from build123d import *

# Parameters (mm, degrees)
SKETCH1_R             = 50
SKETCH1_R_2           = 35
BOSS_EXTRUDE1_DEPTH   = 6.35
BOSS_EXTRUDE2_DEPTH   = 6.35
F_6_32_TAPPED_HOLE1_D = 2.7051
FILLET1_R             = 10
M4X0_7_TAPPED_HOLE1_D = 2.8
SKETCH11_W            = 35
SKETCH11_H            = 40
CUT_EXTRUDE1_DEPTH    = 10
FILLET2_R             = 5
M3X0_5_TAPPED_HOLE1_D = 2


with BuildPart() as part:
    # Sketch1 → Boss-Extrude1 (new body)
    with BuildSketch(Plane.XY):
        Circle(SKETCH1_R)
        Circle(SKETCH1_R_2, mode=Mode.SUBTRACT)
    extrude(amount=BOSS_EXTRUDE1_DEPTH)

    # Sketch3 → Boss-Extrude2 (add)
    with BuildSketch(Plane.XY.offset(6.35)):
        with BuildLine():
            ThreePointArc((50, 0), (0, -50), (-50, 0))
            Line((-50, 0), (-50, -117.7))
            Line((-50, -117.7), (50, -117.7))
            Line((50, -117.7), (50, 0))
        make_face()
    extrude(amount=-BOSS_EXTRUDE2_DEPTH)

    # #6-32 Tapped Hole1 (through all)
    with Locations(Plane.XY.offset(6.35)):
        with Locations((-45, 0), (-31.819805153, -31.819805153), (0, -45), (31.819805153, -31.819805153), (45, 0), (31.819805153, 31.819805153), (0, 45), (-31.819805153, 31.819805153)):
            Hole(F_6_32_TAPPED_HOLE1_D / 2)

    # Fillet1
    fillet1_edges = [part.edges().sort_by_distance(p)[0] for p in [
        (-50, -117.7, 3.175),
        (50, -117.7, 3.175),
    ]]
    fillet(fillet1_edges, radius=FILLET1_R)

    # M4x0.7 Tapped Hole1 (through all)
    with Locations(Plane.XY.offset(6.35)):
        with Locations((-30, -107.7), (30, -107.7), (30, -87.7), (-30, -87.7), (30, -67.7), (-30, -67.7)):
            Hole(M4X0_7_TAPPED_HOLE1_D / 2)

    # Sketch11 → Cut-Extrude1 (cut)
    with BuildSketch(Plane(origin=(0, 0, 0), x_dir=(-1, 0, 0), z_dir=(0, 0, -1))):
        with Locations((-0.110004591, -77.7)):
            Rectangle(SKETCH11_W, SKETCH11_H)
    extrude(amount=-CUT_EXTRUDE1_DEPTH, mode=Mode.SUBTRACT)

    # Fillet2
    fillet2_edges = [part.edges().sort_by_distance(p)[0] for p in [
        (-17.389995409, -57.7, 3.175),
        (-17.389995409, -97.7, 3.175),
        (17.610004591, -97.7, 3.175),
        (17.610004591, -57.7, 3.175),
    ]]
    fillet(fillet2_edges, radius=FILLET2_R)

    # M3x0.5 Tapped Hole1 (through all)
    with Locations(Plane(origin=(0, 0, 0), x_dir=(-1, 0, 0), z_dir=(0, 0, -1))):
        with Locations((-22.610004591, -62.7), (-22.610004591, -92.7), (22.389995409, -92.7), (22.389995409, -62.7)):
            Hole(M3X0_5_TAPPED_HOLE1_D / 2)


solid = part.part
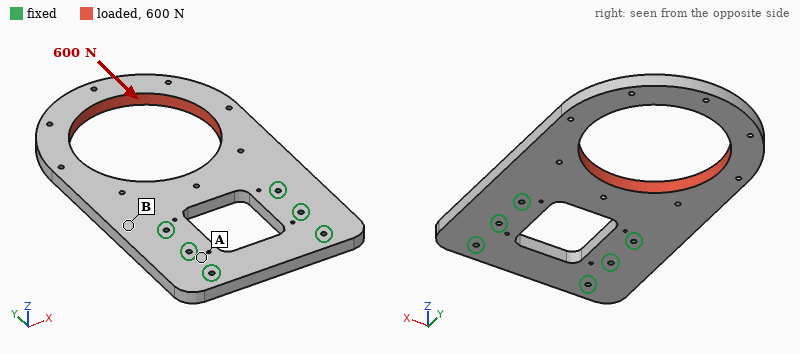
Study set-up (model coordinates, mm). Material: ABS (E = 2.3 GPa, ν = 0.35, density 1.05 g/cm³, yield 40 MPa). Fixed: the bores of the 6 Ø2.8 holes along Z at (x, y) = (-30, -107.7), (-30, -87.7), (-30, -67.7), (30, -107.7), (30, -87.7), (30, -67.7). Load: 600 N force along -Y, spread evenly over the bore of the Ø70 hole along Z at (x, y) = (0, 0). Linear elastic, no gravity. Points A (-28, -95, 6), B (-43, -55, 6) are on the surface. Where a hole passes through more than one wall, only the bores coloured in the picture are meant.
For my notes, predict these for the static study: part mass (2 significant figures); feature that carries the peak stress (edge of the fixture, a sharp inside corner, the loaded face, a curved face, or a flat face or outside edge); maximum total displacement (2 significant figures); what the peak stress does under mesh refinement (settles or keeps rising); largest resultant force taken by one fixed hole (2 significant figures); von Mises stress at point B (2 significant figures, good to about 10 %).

69 g
edge of the fixture
0.19 mm
keeps rising
200 N
1.7 MPa
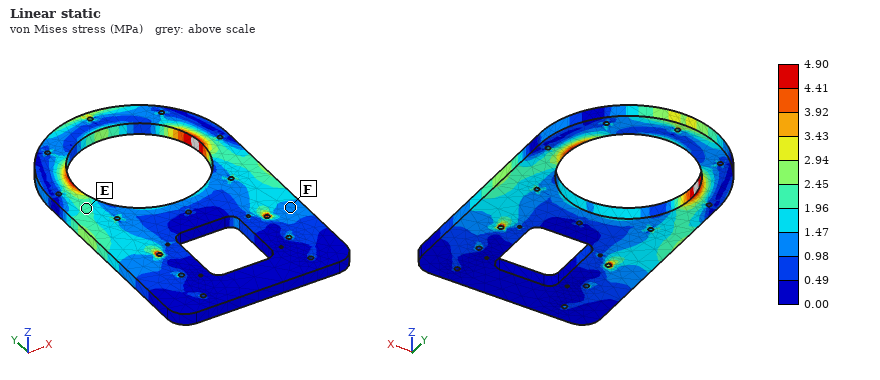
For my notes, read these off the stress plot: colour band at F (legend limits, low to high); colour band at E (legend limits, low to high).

0.98 to 1.47 MPa
1.96 to 2.45 MPa
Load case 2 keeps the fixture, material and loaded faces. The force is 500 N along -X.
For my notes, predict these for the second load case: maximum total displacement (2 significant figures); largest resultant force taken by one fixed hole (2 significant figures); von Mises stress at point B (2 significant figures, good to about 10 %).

0.94 mm
460 N
2.6 MPa
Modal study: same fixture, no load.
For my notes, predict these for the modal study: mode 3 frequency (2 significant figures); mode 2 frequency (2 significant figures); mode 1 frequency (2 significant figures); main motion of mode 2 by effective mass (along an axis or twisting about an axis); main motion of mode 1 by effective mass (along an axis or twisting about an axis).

580 Hz
310 Hz
120 Hz
twisting about Y
along Z
